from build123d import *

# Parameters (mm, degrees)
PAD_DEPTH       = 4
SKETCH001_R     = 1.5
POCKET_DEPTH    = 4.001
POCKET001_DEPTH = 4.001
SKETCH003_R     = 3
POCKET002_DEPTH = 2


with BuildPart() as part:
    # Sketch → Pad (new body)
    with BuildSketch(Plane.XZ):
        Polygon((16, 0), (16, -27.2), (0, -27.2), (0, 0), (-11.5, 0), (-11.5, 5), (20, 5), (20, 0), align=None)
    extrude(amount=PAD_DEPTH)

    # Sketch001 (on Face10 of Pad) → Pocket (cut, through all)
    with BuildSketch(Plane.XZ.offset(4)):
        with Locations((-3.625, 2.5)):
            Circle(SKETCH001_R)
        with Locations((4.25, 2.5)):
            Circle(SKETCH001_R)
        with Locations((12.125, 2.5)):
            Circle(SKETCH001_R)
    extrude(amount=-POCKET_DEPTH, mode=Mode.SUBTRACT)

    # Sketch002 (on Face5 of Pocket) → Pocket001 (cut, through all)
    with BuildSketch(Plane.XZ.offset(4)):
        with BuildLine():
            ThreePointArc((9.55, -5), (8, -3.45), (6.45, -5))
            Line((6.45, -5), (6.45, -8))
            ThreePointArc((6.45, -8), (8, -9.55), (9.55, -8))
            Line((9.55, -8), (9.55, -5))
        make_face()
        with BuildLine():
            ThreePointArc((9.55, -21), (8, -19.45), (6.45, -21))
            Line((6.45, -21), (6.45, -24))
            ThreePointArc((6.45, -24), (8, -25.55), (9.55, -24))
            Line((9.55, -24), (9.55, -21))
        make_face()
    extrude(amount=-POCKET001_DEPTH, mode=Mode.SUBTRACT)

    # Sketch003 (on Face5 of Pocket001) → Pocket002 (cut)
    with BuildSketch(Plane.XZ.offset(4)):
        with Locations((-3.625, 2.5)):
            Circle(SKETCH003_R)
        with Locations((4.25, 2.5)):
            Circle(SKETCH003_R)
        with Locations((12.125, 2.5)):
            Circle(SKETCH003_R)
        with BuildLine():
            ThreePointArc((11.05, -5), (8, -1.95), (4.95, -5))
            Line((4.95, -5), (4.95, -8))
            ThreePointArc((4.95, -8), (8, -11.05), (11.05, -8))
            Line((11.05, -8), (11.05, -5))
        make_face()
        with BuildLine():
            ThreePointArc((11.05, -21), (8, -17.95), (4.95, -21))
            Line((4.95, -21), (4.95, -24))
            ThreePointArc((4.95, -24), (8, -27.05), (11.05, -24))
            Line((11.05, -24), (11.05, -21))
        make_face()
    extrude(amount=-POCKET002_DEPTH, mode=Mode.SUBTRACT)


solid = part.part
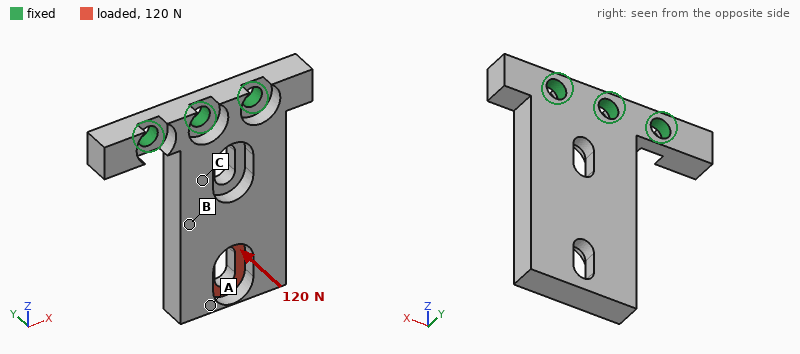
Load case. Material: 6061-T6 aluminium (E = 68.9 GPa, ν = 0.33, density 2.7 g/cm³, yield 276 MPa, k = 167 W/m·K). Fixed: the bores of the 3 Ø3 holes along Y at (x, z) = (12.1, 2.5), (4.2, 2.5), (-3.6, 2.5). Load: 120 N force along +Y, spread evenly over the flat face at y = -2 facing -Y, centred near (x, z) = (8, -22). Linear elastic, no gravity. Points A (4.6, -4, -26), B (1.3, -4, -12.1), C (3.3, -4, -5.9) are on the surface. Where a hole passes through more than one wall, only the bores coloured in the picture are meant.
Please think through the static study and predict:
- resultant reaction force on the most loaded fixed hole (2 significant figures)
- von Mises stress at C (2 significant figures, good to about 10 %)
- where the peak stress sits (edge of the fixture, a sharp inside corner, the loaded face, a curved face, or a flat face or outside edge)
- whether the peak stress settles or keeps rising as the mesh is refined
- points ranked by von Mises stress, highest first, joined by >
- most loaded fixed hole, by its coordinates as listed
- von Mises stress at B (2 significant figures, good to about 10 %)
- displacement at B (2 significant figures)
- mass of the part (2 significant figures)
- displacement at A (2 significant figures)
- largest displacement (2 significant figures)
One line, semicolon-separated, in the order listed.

140 N; 72 MPa; edge of the fixture; keeps rising; C > B > A; (4.2, 2.5); 38 MPa; 0.090 mm; 5.2 g; 0.23 mm; 0.25 mm
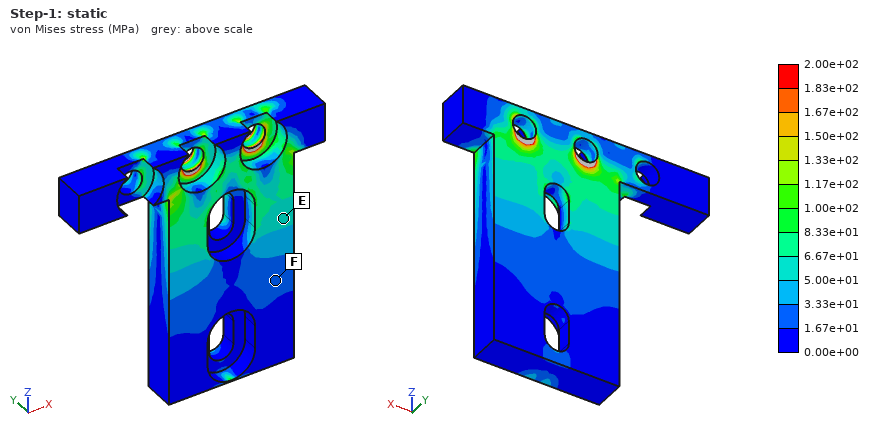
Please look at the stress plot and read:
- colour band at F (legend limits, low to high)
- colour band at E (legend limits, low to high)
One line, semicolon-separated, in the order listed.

1.67e+01 to 3.33e+01 MPa; 5.00e+01 to 6.67e+01 MPa
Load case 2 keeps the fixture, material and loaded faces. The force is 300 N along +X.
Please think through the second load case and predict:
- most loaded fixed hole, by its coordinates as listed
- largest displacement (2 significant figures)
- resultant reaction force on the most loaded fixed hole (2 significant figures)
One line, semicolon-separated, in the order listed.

(12.1, 2.5); 44 µm; 650 N
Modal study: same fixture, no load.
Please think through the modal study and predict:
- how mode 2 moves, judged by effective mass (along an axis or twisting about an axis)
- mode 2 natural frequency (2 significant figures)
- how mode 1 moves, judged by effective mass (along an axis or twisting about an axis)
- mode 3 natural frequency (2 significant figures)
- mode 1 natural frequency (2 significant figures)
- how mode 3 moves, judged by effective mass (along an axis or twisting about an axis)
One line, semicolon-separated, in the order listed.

along X; 10 kHz; along Y; 11 kHz; 3000 Hz; along X
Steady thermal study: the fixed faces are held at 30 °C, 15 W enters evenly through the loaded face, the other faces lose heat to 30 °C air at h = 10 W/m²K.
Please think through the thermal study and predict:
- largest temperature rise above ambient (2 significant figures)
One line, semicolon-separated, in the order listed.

49 K
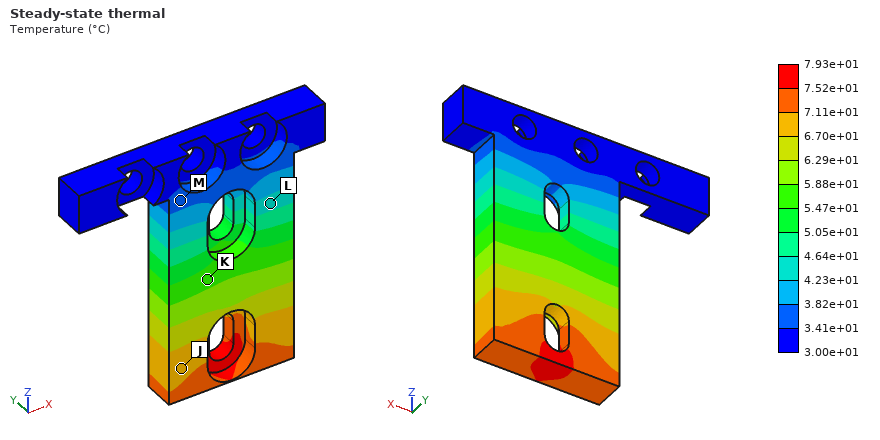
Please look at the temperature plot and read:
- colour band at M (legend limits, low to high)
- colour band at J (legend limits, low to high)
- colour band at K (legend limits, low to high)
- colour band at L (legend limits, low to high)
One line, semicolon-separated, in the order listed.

3.41e+01 to 3.82e+01 °C; 6.70e+01 to 7.11e+01 °C; 5.47e+01 to 5.88e+01 °C; 4.23e+01 to 4.64e+01 °C
